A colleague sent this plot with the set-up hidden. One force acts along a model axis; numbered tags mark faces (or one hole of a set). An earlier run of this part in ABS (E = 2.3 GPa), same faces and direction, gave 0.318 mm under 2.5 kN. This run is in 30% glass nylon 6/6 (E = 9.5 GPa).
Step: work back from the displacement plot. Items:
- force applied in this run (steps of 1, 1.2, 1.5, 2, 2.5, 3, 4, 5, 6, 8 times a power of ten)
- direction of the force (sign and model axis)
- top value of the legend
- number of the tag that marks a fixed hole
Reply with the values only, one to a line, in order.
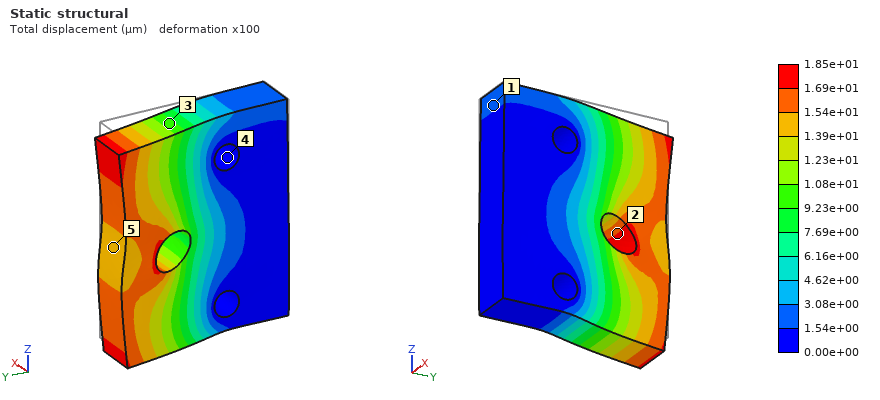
600 N
-Z
1.85e+01 µm
4
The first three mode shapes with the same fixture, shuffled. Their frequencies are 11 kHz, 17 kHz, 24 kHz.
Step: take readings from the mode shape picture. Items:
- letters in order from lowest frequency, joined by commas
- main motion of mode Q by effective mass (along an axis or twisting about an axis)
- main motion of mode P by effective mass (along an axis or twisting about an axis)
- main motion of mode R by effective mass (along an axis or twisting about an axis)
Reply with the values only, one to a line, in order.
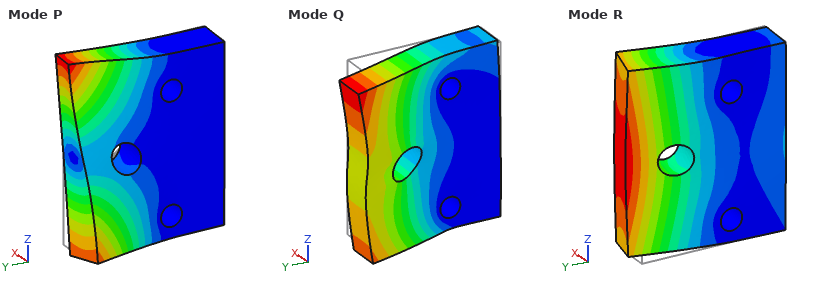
R, P, Q
along Z
twisting about Y
along X
